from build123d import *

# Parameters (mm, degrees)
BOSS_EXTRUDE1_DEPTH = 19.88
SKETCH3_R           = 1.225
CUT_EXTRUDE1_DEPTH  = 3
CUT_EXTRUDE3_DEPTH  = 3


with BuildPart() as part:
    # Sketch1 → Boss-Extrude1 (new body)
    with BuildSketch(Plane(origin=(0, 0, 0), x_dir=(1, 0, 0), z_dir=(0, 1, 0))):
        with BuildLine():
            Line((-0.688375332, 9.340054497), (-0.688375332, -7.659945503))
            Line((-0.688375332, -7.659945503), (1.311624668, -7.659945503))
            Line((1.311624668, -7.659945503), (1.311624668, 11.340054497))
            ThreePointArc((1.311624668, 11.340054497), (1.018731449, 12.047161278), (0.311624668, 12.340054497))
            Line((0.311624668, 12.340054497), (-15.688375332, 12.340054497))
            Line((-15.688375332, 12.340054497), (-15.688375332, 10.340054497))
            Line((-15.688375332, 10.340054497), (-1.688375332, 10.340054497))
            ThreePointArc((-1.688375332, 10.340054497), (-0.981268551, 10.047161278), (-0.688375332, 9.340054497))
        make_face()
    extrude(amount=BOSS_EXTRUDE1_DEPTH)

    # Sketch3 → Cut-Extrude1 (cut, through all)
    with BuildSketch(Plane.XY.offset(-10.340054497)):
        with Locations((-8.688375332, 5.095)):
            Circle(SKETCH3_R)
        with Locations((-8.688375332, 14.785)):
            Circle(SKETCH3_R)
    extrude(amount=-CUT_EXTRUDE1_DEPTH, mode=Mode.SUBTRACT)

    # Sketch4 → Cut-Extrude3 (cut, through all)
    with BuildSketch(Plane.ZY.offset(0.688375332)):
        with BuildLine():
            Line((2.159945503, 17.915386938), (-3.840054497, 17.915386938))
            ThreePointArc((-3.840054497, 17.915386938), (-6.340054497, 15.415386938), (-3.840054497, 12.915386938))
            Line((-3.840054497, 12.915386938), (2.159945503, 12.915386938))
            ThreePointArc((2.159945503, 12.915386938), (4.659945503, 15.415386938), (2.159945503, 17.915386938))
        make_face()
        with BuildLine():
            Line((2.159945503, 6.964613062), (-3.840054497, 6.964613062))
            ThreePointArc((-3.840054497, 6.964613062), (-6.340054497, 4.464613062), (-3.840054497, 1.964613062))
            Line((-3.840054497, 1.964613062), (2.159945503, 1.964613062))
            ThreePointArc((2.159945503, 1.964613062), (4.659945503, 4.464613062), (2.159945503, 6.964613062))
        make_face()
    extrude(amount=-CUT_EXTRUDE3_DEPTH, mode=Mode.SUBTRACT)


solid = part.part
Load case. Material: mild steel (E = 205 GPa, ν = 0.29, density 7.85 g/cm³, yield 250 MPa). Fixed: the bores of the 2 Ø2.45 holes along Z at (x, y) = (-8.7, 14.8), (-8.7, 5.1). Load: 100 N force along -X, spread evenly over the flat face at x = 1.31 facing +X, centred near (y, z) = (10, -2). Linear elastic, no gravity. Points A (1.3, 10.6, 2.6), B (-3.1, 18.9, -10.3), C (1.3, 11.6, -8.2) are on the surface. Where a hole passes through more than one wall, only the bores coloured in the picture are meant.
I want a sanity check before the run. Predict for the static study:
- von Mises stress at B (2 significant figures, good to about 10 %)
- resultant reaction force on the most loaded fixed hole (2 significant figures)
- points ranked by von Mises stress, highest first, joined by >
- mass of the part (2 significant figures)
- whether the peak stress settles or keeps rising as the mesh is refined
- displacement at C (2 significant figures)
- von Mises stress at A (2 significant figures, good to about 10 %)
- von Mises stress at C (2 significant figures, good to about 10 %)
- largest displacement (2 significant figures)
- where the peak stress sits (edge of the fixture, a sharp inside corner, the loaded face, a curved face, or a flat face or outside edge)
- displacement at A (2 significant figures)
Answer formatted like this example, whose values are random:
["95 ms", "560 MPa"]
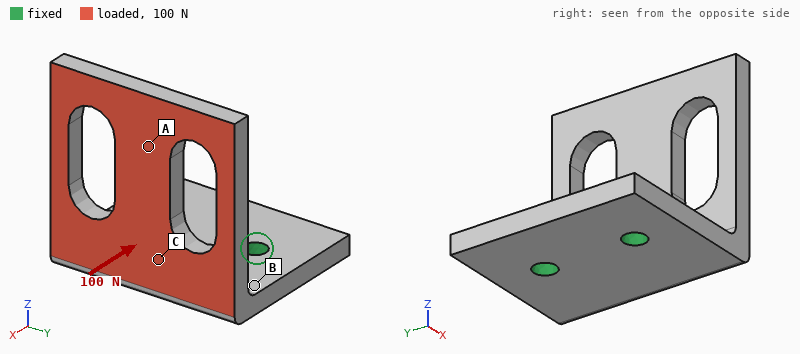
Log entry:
["65 MPa", "51 N", "B > C > A", "9.2 g", "keeps rising", "18 µm", "13 MPa", "51 MPa", "87 µm", "edge of the fixture", "60 µm"]
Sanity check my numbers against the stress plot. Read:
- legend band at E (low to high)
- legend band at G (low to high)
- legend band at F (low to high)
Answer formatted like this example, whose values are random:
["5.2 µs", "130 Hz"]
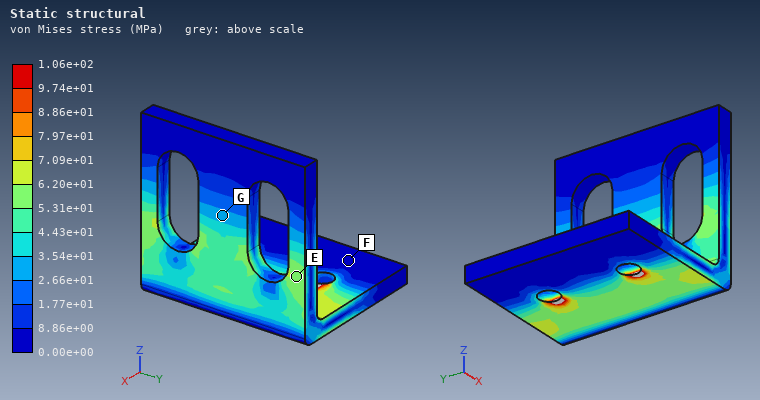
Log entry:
["5.31e+01 to 6.20e+01 MPa", "2.66e+01 to 3.54e+01 MPa", "0.00e+00 to 8.86e+00 MPa"]
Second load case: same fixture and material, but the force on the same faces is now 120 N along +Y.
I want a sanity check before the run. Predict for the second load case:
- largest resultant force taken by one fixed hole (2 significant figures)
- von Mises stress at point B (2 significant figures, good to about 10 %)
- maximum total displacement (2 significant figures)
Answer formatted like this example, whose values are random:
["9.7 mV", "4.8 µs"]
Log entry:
["150 N", "24 MPa", "21 µm"]
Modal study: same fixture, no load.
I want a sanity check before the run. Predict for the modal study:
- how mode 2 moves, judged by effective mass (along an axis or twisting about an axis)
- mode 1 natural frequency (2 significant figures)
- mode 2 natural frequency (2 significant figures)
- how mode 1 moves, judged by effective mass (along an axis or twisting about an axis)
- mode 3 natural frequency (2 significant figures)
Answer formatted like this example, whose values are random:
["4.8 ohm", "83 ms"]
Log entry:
["along Y", "3000 Hz", "6100 Hz", "along X", "9400 Hz"]
